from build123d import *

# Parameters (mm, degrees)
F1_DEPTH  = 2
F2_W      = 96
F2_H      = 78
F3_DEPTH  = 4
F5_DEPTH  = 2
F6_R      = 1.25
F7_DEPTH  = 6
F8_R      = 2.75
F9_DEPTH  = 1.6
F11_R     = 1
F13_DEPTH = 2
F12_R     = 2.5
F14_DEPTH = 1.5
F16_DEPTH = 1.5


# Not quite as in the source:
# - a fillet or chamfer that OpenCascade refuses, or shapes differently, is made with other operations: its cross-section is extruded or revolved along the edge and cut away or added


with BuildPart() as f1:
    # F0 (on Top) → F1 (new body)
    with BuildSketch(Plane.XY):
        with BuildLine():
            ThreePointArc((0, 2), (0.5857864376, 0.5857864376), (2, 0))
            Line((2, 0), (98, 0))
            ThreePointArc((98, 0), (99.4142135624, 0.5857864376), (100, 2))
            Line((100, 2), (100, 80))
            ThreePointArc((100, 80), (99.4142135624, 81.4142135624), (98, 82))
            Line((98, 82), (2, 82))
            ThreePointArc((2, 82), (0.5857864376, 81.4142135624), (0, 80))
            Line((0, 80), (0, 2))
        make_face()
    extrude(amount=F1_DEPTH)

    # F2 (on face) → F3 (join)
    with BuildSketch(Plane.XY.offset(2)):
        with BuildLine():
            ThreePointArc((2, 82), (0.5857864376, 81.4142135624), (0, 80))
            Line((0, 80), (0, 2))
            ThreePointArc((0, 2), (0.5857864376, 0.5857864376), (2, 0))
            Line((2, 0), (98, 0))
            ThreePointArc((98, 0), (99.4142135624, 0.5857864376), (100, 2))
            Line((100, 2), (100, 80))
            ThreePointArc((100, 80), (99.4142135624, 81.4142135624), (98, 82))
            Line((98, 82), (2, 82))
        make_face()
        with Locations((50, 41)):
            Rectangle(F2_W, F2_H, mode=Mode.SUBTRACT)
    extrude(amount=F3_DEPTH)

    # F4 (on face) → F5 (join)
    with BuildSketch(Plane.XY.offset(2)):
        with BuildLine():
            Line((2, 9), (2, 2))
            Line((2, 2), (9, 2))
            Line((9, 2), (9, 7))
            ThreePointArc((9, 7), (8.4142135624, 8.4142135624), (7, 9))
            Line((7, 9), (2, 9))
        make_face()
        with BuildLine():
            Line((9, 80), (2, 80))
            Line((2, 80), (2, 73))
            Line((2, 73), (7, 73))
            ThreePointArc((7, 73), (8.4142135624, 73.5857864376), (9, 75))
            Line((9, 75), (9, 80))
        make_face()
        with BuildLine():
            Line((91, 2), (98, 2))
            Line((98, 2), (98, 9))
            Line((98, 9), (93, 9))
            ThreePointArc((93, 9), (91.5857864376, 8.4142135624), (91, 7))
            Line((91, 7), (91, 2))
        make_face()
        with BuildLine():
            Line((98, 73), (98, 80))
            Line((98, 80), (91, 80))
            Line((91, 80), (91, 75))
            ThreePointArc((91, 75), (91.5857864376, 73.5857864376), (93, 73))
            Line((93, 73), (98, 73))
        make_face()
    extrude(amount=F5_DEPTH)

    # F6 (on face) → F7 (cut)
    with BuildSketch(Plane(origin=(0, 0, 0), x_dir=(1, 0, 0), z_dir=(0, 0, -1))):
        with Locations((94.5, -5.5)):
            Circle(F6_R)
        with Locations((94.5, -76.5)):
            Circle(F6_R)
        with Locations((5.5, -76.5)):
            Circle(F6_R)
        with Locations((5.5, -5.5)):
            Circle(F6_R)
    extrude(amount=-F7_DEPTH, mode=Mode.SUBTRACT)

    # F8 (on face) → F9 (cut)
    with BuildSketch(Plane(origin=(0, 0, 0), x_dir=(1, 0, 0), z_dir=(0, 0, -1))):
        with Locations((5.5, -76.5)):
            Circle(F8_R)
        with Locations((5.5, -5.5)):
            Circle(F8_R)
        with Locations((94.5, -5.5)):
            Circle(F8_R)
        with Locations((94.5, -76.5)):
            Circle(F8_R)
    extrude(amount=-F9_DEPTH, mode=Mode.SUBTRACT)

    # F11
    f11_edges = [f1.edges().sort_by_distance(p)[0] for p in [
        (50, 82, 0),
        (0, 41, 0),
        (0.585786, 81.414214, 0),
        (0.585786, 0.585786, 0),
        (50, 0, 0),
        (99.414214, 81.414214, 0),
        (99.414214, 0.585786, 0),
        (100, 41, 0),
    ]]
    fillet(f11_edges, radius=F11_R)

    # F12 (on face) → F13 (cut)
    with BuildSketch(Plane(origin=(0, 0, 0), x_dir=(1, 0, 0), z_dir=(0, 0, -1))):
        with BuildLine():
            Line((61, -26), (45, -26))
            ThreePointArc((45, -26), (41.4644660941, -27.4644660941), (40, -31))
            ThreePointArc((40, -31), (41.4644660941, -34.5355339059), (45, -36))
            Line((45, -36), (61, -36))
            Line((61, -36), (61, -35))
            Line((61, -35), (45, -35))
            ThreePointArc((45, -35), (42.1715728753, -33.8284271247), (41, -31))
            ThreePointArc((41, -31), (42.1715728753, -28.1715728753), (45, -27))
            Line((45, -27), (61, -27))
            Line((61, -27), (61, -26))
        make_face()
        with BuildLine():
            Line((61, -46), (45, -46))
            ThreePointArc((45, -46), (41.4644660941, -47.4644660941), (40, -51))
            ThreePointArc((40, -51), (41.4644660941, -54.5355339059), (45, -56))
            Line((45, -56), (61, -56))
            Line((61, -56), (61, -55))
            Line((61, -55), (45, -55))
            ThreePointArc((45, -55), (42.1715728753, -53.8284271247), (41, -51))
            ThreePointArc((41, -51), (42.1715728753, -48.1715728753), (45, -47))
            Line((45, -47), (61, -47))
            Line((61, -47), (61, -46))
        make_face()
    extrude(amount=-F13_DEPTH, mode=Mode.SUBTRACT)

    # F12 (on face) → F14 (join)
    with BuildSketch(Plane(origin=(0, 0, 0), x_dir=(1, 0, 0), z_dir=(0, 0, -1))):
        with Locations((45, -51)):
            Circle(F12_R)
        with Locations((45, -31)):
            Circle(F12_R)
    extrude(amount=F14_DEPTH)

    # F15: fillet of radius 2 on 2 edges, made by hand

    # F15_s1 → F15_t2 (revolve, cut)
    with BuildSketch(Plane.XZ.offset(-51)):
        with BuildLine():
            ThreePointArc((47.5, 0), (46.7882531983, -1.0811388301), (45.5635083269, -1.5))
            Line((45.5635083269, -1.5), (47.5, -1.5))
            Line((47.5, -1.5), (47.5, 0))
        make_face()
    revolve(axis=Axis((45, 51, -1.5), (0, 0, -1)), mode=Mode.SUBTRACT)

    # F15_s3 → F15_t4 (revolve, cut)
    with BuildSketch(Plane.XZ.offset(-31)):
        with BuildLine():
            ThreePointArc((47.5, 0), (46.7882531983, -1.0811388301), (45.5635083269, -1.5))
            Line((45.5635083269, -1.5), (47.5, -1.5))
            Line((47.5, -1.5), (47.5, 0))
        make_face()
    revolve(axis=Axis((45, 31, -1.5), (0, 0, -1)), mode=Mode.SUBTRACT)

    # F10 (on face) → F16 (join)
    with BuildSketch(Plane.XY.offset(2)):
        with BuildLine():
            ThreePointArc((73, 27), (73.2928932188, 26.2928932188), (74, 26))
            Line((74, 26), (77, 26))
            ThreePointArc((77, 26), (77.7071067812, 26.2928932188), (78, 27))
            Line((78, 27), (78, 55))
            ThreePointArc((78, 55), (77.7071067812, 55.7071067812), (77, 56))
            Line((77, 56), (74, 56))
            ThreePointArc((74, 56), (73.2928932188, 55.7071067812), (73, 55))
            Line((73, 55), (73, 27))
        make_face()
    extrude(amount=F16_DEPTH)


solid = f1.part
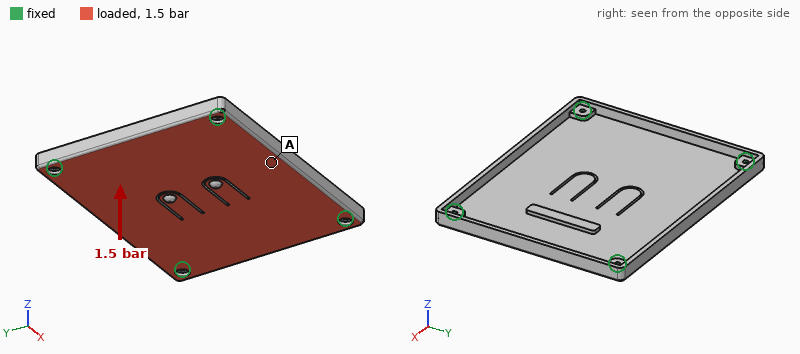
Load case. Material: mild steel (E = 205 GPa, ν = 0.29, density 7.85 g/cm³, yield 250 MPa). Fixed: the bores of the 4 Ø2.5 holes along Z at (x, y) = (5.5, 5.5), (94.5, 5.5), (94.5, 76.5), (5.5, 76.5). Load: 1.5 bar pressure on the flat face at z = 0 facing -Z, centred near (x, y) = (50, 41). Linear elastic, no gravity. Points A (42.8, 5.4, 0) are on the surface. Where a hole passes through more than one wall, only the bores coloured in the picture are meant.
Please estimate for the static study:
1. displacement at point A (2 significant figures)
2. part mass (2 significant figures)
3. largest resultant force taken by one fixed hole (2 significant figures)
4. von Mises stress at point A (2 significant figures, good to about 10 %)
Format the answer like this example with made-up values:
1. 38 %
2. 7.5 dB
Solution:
1. 0.090 mm
2. 150 g
3. 660 N
4. 46 MPa
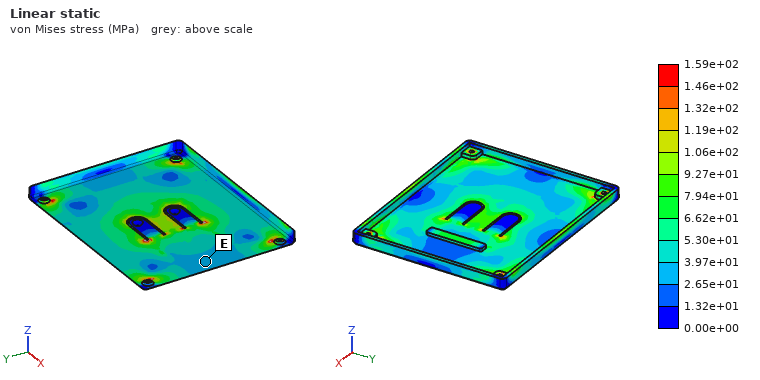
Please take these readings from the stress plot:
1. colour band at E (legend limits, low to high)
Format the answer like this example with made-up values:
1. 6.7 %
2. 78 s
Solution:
1. 2.65e+01 to 3.97e+01 MPa
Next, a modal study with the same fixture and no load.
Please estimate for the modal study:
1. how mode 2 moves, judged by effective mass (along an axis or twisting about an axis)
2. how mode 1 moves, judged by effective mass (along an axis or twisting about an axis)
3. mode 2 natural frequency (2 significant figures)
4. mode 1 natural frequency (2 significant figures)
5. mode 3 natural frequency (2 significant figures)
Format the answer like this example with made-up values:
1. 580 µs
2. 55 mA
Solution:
1. twisting about X
2. along Z
3. 2200 Hz
4. 1200 Hz
5. 2600 Hz
